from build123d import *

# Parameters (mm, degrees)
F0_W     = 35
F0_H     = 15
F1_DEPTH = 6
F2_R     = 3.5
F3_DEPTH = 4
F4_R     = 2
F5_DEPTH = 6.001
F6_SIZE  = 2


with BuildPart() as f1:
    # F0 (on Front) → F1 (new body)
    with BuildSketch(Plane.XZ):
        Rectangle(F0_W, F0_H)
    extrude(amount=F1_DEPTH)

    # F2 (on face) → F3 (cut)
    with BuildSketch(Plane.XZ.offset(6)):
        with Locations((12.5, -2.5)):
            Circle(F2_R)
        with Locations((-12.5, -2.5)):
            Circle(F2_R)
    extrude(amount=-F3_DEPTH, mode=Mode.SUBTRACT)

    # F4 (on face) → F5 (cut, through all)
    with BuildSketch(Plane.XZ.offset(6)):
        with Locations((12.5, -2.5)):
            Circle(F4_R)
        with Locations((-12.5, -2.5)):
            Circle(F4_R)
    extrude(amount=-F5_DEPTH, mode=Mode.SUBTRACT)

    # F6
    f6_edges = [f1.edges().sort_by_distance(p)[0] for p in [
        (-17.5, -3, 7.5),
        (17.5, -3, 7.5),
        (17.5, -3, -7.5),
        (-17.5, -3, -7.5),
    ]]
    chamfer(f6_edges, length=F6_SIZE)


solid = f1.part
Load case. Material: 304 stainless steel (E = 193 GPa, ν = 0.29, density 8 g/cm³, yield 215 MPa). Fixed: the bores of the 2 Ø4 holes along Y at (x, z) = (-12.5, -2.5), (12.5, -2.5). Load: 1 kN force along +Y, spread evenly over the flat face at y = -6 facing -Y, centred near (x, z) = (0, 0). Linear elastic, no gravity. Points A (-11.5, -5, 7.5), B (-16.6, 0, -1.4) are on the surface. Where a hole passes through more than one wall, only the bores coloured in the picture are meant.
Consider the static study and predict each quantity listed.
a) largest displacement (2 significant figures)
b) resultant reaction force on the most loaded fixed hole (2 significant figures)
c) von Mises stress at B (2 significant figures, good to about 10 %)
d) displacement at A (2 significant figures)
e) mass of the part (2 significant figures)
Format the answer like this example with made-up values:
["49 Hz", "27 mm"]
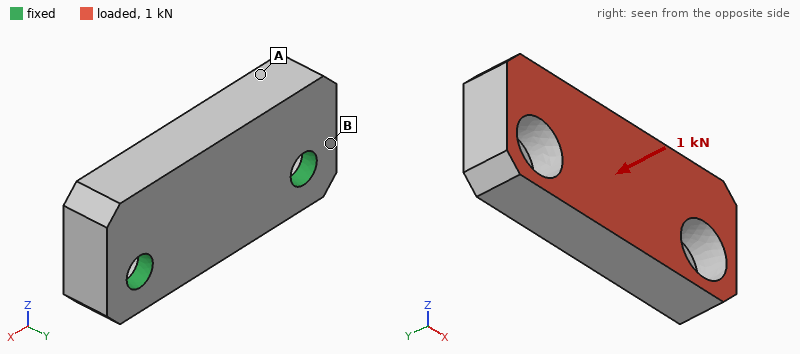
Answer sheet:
["7.9 µm", "540 N", "23 MPa", "6.4 µm", "22 g"]
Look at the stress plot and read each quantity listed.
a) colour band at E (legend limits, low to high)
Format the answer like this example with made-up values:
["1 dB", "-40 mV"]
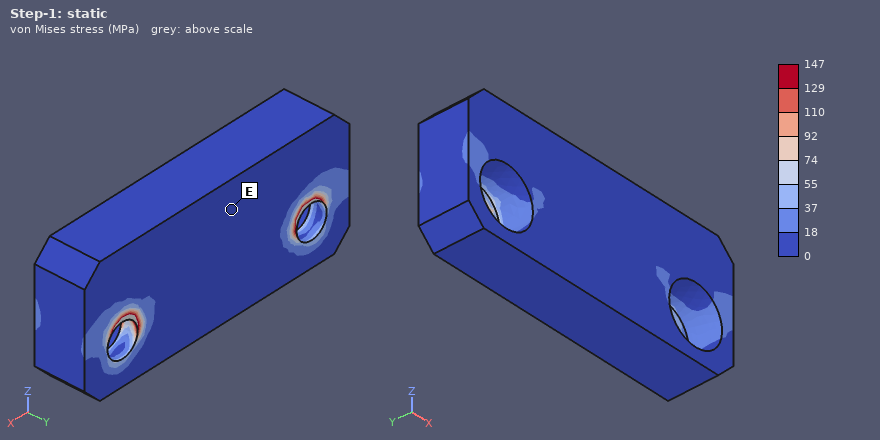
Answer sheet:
["0 to 18 MPa"]
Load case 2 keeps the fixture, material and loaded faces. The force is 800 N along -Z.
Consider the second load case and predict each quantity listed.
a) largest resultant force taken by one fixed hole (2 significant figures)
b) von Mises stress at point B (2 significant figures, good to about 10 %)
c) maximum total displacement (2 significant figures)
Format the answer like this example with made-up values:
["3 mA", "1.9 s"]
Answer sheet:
["410 N", "22 MPa", "9.1 µm"]
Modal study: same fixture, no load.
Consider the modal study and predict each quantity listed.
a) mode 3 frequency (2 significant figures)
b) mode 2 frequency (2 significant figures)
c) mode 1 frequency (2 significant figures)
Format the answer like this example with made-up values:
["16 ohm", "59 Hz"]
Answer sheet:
["28 kHz", "28 kHz", "14 kHz"]
